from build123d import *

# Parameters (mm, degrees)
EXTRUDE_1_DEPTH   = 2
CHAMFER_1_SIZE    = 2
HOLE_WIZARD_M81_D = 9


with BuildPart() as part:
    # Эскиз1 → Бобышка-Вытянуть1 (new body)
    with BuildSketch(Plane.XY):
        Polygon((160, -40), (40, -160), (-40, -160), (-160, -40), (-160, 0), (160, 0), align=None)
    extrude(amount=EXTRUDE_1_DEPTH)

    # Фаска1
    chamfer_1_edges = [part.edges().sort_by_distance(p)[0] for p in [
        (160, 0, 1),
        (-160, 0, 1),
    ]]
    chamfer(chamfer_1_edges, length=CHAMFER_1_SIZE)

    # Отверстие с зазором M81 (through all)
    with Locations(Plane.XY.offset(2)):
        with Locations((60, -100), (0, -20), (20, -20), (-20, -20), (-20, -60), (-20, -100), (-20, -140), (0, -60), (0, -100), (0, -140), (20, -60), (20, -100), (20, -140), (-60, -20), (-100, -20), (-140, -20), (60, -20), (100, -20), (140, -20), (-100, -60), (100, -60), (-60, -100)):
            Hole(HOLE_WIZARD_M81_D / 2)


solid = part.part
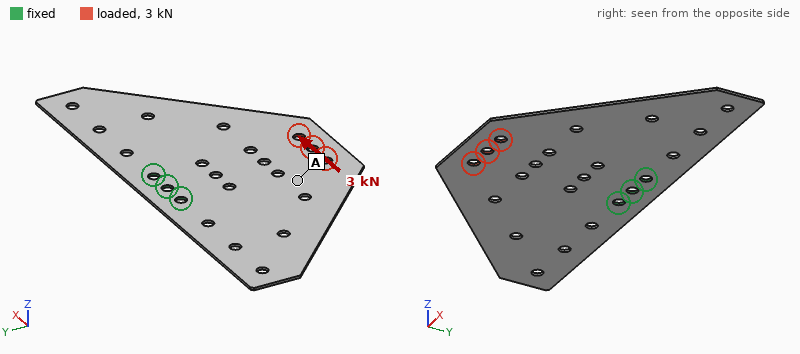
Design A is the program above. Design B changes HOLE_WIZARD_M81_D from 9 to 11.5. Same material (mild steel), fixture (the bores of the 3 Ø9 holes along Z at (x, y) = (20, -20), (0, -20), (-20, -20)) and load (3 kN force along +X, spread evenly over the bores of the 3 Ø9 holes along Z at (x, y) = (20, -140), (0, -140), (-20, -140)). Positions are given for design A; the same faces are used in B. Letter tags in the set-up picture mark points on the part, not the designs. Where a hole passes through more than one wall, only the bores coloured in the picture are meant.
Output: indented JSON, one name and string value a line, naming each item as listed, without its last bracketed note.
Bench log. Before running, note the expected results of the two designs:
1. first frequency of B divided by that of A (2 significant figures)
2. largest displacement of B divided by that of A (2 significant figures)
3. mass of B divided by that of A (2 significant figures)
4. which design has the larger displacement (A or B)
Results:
{
  "first frequency of B divided by that of A": "1.0",
  "largest displacement of B divided by that of A": "0.92",
  "mass of B divided by that of A": "0.97",
  "which design has the larger displacement": "A"
}
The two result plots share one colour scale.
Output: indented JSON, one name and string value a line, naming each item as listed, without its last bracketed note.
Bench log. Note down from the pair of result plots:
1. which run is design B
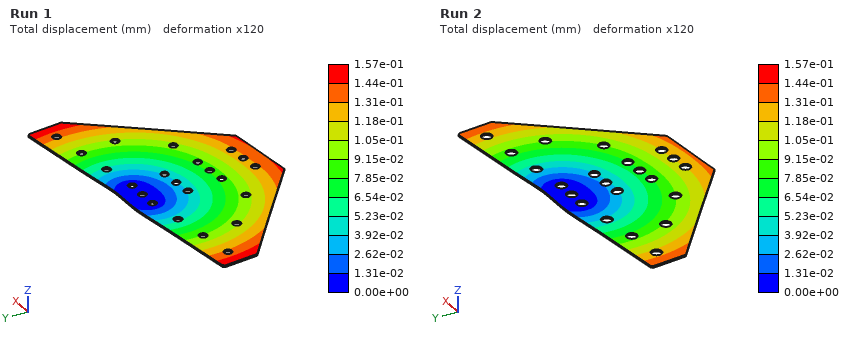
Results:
{
  "which run is design B": "Run 2"
}
